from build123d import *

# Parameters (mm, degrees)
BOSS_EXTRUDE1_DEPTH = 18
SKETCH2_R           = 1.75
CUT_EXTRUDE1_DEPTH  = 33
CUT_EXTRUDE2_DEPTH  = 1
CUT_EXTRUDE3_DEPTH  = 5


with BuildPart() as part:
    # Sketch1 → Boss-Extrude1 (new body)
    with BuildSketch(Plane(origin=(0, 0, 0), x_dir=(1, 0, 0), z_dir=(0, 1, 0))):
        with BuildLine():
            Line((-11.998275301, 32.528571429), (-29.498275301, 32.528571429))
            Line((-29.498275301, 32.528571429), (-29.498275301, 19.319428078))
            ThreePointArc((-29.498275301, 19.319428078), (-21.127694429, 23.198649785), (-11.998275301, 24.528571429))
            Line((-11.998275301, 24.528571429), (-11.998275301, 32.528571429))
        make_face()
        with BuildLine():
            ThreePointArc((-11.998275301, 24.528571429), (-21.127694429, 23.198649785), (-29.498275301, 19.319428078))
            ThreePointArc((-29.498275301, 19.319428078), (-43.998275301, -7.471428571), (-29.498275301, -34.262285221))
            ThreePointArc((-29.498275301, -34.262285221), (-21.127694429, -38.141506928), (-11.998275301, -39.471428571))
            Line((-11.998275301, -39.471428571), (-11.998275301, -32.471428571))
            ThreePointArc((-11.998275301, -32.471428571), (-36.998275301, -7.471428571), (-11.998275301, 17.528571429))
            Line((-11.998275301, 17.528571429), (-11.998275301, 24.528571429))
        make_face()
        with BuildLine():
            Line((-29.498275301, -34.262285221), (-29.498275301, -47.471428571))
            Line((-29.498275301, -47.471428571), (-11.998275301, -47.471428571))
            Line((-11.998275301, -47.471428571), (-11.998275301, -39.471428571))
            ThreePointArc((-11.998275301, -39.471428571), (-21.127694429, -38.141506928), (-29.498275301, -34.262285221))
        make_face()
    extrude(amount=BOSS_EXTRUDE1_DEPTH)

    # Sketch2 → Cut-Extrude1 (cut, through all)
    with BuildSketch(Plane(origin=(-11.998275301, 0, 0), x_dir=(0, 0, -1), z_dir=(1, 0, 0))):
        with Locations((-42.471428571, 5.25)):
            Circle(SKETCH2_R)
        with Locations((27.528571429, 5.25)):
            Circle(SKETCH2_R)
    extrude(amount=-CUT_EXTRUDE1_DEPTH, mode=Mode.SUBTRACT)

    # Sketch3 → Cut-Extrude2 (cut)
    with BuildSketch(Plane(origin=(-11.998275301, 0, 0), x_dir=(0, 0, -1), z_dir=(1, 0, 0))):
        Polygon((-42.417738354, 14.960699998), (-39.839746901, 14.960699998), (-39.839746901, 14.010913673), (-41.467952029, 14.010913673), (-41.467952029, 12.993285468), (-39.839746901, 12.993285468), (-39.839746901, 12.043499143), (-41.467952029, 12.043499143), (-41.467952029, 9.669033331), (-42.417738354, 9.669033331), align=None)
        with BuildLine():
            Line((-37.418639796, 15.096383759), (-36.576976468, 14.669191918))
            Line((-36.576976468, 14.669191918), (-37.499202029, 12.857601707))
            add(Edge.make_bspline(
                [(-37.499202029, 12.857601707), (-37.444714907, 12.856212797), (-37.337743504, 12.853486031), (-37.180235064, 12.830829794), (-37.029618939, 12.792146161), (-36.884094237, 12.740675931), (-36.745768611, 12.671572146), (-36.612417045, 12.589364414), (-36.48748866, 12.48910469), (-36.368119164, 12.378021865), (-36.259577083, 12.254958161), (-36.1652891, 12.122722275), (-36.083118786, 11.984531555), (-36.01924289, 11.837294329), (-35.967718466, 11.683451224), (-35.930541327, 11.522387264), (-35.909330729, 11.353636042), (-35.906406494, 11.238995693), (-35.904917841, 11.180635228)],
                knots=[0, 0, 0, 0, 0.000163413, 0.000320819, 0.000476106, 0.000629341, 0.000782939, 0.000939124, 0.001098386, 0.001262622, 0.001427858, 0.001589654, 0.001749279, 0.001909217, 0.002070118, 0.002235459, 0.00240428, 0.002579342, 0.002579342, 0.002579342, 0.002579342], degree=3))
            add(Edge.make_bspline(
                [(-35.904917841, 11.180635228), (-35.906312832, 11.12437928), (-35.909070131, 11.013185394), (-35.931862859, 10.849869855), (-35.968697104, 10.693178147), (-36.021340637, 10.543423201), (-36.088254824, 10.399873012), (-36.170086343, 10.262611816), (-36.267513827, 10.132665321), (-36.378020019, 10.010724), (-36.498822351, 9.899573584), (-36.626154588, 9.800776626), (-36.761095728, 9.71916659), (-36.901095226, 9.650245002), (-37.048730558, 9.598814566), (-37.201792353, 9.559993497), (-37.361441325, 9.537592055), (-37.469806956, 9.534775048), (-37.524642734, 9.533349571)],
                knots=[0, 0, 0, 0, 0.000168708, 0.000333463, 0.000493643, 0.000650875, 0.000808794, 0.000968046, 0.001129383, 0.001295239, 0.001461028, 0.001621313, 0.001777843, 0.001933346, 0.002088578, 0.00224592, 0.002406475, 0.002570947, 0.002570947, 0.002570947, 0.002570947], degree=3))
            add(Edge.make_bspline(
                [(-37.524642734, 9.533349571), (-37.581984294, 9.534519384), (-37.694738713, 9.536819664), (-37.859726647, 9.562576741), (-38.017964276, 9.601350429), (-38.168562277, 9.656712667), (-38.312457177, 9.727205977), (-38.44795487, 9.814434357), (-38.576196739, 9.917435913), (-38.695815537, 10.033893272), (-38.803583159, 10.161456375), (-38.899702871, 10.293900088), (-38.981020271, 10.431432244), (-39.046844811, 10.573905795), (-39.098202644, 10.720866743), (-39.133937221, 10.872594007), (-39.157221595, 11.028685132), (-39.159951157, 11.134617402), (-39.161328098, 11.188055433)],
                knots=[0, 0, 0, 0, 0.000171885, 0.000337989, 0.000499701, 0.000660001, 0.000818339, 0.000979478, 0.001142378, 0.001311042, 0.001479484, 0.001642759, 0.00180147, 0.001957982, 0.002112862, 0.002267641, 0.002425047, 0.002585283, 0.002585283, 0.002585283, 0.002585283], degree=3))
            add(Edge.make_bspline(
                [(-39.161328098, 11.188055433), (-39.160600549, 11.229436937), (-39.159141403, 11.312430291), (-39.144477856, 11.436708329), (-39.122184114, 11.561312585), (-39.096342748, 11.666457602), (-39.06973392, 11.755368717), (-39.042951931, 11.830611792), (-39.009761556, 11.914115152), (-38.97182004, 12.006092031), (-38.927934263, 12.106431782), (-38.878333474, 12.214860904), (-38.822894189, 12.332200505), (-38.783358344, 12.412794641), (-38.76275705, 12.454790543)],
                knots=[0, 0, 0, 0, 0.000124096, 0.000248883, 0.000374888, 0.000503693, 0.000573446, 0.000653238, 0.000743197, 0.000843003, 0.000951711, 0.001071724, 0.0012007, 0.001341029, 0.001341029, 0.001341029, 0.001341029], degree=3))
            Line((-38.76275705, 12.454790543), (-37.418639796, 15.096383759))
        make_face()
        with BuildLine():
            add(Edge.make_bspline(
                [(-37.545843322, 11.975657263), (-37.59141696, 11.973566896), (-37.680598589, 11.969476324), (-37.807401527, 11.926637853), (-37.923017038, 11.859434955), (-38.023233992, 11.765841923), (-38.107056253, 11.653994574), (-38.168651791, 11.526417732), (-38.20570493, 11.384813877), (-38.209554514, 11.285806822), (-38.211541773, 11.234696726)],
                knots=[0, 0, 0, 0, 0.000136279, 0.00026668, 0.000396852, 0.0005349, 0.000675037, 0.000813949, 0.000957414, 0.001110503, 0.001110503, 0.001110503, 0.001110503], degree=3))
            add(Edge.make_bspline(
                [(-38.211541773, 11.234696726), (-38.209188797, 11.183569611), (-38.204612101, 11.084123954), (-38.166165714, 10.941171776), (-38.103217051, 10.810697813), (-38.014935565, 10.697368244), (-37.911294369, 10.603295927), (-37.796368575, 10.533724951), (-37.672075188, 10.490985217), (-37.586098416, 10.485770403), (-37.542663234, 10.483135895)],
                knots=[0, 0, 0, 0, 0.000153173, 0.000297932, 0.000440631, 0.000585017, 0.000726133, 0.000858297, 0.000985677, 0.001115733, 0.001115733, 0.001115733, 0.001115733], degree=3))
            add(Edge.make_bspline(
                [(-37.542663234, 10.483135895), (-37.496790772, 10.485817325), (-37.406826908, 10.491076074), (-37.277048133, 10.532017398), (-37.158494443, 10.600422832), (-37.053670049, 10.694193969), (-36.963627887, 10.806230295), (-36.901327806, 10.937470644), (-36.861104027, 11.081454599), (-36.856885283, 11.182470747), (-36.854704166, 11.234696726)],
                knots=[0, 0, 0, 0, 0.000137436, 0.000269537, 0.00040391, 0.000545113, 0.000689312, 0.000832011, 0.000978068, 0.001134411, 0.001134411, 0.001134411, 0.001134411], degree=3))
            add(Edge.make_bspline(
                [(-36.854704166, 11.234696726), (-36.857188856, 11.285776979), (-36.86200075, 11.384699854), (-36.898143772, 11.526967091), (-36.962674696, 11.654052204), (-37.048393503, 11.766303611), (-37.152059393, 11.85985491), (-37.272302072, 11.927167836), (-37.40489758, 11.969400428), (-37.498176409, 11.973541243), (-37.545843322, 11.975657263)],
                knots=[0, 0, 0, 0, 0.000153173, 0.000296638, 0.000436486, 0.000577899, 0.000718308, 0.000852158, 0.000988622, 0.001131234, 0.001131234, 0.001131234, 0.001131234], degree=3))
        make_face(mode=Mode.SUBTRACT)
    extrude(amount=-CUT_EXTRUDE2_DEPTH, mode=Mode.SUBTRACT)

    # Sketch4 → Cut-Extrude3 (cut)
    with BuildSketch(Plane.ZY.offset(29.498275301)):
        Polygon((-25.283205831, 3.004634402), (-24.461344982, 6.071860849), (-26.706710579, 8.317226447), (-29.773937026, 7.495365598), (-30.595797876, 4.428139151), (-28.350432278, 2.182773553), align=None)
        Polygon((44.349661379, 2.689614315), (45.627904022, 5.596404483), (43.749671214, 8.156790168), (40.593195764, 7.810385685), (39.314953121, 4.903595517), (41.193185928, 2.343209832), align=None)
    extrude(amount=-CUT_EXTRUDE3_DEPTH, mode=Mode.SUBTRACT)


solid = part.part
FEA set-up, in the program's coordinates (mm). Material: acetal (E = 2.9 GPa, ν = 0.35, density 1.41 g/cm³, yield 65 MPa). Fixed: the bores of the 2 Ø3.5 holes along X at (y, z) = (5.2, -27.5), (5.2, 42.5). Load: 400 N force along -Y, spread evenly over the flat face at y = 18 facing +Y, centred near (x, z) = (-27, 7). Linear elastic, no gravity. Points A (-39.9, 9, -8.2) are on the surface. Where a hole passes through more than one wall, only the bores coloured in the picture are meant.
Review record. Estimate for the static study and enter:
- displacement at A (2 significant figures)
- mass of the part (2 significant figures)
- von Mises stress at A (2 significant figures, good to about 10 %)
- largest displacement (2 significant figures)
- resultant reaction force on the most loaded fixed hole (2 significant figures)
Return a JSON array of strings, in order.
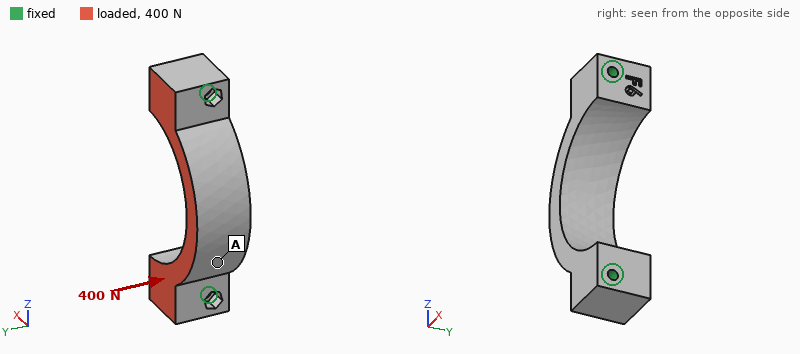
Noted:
["0.13 mm", "24 g", "2.9 MPa", "0.18 mm", "200 N"]
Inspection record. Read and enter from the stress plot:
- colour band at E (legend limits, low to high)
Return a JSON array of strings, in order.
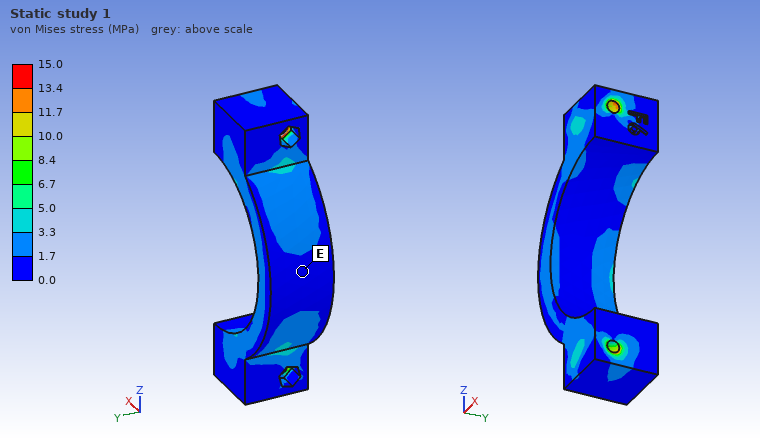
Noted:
["0.0 to 1.7 MPa"]
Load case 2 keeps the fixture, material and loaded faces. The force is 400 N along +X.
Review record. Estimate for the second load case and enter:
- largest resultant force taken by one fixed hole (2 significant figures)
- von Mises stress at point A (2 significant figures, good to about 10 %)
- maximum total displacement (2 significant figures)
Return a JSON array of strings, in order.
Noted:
["210 N", "1.9 MPa", "0.15 mm"]
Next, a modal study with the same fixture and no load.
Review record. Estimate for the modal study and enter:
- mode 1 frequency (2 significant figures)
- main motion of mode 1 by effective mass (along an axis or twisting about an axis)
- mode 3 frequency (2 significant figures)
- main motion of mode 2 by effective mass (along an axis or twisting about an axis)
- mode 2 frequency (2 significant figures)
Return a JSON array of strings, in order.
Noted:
["1900 Hz", "along Y", "4900 Hz", "along Z", "3700 Hz"]
